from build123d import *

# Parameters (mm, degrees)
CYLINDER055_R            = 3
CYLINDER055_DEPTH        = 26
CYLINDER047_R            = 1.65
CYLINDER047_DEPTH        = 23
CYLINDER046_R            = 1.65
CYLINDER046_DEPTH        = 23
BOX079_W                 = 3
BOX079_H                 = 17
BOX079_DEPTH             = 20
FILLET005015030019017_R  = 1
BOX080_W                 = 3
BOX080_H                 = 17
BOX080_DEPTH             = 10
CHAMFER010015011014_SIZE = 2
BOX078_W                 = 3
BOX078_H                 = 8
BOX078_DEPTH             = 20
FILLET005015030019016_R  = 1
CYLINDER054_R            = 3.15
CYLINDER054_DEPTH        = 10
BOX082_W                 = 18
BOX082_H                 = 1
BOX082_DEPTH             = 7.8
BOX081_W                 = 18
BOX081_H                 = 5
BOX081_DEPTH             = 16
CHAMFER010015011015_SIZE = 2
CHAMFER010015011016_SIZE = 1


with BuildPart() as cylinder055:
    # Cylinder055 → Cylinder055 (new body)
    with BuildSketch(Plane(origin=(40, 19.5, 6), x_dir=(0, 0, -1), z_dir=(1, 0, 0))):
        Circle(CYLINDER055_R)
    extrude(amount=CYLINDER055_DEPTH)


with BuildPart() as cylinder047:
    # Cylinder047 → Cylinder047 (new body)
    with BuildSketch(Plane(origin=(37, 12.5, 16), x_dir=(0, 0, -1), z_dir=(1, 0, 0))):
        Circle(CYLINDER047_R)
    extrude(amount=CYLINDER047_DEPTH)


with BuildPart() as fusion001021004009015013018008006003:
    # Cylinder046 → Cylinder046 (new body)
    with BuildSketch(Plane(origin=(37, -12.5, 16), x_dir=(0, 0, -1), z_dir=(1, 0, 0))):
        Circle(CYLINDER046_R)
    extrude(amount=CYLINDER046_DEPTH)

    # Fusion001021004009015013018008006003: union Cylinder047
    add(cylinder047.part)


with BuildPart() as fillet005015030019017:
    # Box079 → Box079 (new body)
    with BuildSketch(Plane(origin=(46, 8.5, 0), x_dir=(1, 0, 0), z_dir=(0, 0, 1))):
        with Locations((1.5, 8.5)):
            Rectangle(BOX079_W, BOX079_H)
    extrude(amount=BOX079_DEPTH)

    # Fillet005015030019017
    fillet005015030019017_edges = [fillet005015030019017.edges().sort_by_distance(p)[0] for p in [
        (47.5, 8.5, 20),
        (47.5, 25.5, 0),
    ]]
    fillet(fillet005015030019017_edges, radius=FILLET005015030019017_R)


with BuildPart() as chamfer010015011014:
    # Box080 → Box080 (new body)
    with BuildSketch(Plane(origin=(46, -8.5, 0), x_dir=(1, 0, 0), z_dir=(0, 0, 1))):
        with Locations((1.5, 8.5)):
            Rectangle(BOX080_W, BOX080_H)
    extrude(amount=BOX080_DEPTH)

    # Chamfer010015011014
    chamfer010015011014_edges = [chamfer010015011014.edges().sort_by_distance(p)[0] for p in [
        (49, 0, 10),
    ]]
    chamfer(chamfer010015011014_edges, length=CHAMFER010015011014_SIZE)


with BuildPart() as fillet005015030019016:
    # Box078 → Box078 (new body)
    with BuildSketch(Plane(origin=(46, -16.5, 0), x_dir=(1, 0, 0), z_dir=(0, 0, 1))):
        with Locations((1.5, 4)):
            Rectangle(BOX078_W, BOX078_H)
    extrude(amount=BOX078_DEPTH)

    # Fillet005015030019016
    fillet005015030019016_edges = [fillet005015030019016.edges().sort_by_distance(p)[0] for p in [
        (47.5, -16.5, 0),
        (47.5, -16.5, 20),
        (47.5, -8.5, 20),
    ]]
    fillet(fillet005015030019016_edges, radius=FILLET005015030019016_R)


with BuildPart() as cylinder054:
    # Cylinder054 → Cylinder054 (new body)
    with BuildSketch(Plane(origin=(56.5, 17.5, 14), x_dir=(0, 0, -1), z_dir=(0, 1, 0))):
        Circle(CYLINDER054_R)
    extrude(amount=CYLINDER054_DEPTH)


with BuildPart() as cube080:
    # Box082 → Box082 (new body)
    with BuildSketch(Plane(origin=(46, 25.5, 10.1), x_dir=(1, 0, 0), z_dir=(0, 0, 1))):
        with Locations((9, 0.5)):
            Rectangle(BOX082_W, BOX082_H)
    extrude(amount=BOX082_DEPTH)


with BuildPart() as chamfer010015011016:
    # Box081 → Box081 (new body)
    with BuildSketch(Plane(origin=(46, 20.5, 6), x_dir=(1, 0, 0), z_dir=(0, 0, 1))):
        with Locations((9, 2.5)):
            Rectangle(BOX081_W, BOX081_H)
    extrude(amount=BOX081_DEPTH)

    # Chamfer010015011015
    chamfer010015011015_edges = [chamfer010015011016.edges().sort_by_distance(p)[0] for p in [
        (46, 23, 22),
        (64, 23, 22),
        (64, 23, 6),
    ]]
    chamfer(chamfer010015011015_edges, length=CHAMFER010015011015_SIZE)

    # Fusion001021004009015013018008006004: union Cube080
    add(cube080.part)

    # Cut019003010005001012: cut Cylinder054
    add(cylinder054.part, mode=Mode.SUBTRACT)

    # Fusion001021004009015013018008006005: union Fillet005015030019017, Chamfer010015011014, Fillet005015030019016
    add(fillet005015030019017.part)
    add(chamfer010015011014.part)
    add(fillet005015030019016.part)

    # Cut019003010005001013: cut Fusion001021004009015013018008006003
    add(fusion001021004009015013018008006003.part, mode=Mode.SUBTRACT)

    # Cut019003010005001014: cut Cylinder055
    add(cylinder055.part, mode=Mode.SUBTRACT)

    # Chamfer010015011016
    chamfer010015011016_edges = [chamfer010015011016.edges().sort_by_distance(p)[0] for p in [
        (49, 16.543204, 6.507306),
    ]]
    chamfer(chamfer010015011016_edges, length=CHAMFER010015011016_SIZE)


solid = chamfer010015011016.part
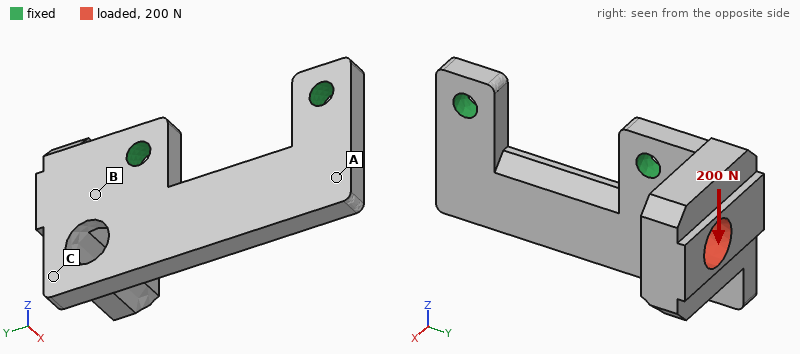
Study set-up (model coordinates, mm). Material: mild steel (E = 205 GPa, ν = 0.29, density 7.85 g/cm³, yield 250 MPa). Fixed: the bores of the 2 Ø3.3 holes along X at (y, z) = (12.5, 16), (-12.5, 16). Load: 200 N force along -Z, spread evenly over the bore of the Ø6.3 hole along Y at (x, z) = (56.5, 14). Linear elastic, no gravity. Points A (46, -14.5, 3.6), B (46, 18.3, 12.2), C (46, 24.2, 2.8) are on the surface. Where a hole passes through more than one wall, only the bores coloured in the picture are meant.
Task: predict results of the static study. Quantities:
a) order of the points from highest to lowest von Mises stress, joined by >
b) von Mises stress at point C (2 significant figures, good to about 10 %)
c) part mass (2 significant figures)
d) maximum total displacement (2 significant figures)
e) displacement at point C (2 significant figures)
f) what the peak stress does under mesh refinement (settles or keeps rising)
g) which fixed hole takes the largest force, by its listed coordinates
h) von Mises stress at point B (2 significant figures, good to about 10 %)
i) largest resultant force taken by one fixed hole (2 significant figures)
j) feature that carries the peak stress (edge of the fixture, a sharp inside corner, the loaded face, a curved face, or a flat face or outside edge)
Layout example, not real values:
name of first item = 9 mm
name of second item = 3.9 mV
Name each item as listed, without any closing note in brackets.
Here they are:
order of the points from highest to lowest von Mises stress, joined by > = B > C > A
von Mises stress at point C = 21 MPa
part mass = 23 g
maximum total displacement = 30 µm
displacement at point C = 18 µm
what the peak stress does under mesh refinement = keeps rising
which fixed hole takes the largest force, by its listed coordinates = (12.5, 16)
von Mises stress at point B = 36 MPa
largest resultant force taken by one fixed hole = 250 N
feature that carries the peak stress = edge of the fixture
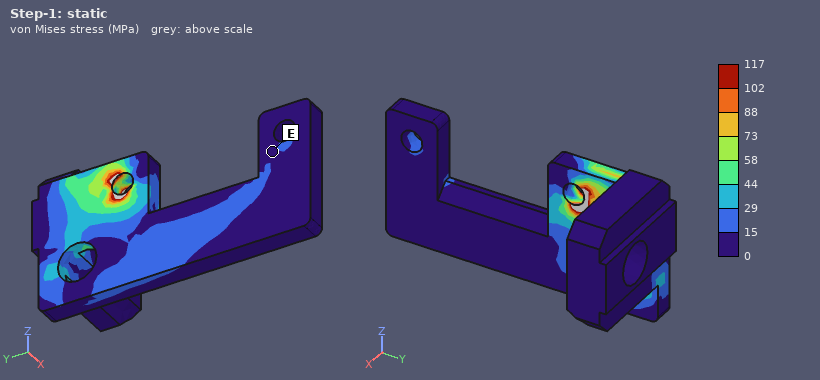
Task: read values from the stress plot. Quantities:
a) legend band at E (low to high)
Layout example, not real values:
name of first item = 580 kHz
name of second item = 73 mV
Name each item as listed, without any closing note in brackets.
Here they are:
legend band at E = 0 to 15 MPa
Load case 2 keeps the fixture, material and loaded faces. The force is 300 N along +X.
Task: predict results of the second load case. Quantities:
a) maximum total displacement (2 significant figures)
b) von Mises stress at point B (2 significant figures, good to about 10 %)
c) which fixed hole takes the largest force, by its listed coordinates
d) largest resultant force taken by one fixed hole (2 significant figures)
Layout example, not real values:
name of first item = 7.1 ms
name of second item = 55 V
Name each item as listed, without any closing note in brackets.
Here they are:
maximum total displacement = 52 µm
von Mises stress at point B = 66 MPa
which fixed hole takes the largest force, by its listed coordinates = (12.5, 16)
largest resultant force taken by one fixed hole = 320 N
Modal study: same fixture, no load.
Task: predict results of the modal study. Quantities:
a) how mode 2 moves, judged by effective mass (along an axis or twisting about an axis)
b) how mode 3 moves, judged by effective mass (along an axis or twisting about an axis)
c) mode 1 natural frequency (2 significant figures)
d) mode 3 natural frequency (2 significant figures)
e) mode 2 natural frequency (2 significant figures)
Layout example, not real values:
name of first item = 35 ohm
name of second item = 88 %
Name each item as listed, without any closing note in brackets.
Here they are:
how mode 2 moves, judged by effective mass = along Z
how mode 3 moves, judged by effective mass = along X
mode 1 natural frequency = 3700 Hz
mode 3 natural frequency = 8100 Hz
mode 2 natural frequency = 4800 Hz
